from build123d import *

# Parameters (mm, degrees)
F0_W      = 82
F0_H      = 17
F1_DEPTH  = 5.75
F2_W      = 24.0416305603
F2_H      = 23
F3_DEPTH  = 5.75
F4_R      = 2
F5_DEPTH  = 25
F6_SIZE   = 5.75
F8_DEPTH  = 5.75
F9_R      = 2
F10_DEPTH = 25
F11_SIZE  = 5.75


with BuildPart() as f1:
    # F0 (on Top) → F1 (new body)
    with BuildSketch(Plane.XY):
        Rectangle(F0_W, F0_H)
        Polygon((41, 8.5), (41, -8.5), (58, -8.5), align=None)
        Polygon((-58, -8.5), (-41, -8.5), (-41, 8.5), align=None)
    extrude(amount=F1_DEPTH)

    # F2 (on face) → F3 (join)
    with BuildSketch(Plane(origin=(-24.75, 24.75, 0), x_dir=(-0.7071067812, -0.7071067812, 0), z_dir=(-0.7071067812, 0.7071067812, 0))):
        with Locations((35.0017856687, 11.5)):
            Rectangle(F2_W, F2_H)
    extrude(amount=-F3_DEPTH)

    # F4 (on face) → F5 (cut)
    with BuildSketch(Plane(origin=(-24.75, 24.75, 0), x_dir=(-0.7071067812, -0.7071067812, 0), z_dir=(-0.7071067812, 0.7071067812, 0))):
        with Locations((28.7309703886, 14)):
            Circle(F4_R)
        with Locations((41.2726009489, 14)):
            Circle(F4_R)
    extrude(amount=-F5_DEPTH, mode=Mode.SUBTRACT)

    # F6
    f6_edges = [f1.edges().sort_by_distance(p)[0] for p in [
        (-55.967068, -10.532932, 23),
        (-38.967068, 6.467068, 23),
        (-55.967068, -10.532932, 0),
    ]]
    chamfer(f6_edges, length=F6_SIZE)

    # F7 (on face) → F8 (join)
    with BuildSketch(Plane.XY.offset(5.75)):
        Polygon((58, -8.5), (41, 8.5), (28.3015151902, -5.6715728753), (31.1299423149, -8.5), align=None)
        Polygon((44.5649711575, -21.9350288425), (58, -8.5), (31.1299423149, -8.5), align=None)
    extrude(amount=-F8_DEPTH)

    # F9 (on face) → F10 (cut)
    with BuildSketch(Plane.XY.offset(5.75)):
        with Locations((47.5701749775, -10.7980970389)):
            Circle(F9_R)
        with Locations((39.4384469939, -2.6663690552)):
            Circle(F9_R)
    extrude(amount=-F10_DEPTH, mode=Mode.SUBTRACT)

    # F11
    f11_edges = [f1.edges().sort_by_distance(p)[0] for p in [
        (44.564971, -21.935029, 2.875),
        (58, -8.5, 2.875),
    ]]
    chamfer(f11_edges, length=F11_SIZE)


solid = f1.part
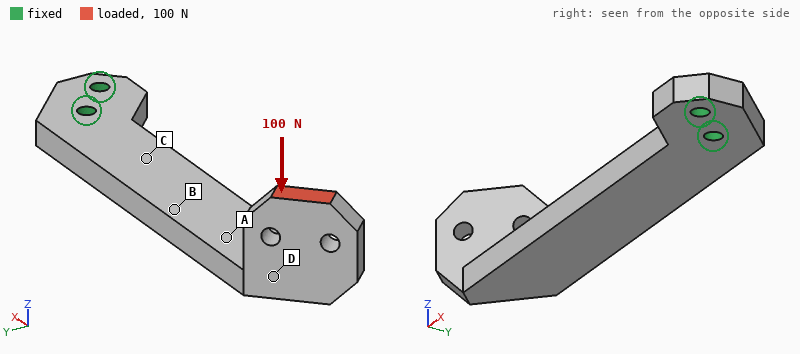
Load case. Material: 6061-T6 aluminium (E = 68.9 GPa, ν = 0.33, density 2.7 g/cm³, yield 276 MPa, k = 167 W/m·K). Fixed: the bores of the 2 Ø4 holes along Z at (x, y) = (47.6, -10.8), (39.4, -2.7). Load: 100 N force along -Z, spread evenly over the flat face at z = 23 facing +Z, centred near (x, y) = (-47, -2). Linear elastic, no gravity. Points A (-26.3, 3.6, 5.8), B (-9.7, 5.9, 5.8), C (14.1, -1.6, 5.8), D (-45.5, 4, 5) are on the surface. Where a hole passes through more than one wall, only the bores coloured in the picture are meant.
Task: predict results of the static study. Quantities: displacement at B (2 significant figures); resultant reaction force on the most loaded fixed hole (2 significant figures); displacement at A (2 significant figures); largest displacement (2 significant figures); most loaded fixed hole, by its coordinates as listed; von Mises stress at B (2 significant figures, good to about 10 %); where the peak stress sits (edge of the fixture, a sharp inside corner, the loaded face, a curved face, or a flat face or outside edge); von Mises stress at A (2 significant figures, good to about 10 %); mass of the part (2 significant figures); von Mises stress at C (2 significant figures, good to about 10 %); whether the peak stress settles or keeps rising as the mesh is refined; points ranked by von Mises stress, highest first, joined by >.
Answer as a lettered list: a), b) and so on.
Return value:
a) 0.45 mm
b) 280 N
c) 0.74 mm
d) 1.4 mm
e) (39.4, -2.7)
f) 40 MPa
g) edge of the fixture
h) 23 MPa
i) 34 g
j) 66 MPa
k) keeps rising
l) C > B > A > D
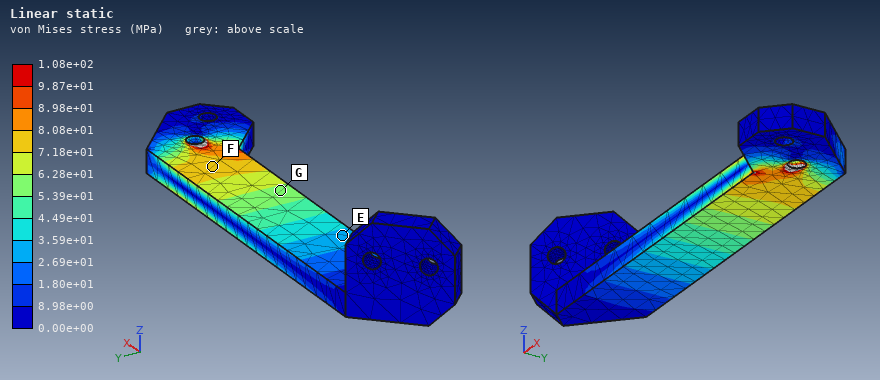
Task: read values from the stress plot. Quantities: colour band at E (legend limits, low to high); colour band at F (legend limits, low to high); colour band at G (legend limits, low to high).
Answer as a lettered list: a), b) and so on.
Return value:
a) 2.69e+01 to 3.59e+01 MPa
b) 7.18e+01 to 8.08e+01 MPa
c) 5.39e+01 to 6.28e+01 MPa
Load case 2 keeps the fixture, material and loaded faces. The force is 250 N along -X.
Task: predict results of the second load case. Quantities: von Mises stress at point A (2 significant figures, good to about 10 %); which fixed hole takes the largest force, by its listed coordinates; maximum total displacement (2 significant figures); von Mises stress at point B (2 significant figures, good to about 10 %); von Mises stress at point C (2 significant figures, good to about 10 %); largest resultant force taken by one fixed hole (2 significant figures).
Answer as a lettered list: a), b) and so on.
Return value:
a) 56 MPa
b) (39.4, -2.7)
c) 1.3 mm
d) 55 MPa
e) 56 MPa
f) 250 N
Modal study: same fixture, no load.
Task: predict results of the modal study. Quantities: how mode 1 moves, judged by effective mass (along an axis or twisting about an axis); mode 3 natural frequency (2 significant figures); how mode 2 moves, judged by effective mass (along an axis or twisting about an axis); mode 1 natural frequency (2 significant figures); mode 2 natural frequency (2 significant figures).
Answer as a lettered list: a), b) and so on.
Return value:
a) along Z
b) 2600 Hz
c) along Y
d) 430 Hz
e) 1100 Hz
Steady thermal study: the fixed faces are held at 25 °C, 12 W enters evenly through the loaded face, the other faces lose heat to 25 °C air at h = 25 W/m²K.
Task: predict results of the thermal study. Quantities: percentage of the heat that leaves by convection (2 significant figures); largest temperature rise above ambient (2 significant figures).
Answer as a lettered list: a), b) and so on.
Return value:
a) 31 %
b) 59 K
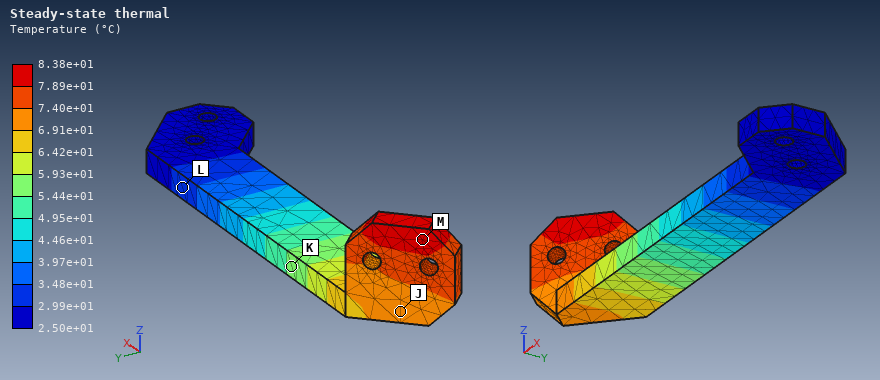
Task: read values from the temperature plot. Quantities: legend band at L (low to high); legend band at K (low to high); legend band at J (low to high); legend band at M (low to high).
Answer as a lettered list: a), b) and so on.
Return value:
a) 2.99e+01 to 3.48e+01 °C
b) 5.44e+01 to 5.93e+01 °C
c) 6.91e+01 to 7.40e+01 °C
d) 7.89e+01 to 8.38e+01 °C
